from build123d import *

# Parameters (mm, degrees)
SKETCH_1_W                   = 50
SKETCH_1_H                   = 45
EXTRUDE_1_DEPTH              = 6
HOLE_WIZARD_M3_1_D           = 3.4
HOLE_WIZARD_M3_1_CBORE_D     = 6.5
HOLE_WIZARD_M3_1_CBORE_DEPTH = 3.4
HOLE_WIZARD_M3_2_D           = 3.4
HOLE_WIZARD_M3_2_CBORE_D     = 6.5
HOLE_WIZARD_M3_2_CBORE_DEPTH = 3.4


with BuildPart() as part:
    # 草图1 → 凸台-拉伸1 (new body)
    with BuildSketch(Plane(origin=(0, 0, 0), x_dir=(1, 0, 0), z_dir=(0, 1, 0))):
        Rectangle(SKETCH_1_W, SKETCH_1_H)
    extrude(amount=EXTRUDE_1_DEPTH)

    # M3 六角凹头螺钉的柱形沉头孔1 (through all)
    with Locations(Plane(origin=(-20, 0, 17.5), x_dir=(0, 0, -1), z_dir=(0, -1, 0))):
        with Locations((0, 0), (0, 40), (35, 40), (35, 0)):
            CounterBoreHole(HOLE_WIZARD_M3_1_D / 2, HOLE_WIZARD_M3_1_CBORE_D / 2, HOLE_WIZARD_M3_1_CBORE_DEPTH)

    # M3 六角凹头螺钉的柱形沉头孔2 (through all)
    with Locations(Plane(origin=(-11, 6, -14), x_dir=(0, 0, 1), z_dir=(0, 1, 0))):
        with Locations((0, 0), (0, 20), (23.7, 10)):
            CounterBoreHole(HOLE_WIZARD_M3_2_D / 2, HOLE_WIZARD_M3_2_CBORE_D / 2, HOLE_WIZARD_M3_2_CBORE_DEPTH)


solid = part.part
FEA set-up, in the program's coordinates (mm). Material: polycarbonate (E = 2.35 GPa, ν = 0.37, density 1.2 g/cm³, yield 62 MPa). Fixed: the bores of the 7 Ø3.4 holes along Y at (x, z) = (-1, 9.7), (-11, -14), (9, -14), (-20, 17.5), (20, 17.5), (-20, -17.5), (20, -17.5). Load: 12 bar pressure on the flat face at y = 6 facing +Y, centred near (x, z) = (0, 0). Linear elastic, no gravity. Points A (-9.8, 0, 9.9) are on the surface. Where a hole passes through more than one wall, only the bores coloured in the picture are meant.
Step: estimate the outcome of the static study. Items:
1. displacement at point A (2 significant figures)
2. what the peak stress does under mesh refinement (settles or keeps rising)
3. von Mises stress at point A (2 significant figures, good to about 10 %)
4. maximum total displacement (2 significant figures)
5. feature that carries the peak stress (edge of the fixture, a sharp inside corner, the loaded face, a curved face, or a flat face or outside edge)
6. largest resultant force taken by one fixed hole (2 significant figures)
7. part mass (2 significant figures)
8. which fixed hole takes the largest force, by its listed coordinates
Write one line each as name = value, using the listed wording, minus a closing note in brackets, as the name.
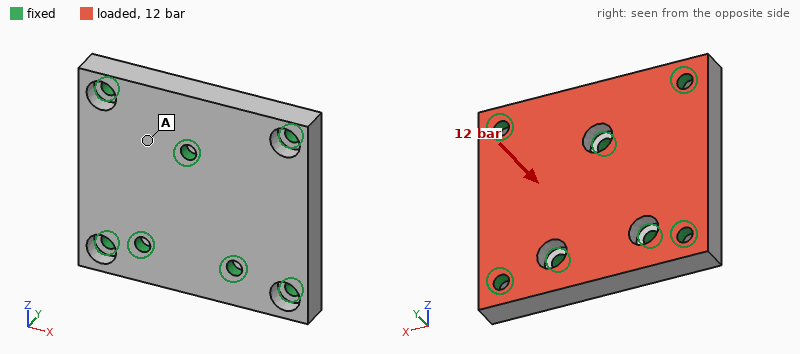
displacement at point A = 0.086 mm
what the peak stress does under mesh refinement = keeps rising
von Mises stress at point A = 5.2 MPa
maximum total displacement = 0.22 mm
feature that carries the peak stress = edge of the fixture
largest resultant force taken by one fixed hole = 620 N
part mass = 15 g
which fixed hole takes the largest force, by its listed coordinates = (-1, 9.7)
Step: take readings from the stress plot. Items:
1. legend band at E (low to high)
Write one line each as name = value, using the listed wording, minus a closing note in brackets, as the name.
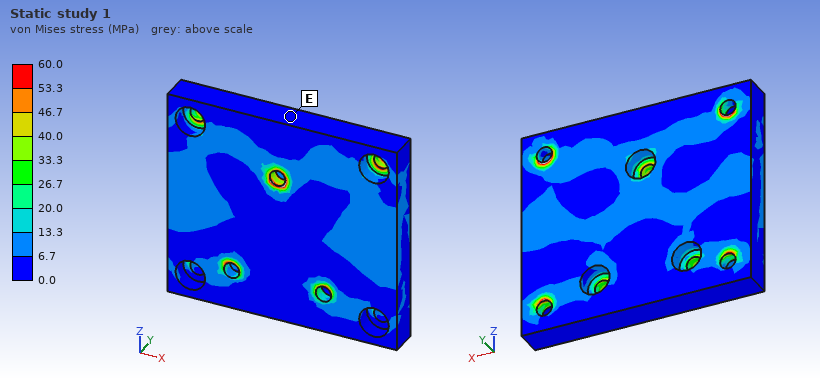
legend band at E = 0.0 to 6.7 MPa
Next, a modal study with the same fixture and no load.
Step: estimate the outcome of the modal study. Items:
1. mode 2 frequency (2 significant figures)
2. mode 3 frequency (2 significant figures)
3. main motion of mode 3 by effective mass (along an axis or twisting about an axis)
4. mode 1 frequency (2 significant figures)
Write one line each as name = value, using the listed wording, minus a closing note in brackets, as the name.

mode 2 frequency = 5500 Hz
mode 3 frequency = 6700 Hz
main motion of mode 3 by effective mass = along Y
mode 1 frequency = 5300 Hz
